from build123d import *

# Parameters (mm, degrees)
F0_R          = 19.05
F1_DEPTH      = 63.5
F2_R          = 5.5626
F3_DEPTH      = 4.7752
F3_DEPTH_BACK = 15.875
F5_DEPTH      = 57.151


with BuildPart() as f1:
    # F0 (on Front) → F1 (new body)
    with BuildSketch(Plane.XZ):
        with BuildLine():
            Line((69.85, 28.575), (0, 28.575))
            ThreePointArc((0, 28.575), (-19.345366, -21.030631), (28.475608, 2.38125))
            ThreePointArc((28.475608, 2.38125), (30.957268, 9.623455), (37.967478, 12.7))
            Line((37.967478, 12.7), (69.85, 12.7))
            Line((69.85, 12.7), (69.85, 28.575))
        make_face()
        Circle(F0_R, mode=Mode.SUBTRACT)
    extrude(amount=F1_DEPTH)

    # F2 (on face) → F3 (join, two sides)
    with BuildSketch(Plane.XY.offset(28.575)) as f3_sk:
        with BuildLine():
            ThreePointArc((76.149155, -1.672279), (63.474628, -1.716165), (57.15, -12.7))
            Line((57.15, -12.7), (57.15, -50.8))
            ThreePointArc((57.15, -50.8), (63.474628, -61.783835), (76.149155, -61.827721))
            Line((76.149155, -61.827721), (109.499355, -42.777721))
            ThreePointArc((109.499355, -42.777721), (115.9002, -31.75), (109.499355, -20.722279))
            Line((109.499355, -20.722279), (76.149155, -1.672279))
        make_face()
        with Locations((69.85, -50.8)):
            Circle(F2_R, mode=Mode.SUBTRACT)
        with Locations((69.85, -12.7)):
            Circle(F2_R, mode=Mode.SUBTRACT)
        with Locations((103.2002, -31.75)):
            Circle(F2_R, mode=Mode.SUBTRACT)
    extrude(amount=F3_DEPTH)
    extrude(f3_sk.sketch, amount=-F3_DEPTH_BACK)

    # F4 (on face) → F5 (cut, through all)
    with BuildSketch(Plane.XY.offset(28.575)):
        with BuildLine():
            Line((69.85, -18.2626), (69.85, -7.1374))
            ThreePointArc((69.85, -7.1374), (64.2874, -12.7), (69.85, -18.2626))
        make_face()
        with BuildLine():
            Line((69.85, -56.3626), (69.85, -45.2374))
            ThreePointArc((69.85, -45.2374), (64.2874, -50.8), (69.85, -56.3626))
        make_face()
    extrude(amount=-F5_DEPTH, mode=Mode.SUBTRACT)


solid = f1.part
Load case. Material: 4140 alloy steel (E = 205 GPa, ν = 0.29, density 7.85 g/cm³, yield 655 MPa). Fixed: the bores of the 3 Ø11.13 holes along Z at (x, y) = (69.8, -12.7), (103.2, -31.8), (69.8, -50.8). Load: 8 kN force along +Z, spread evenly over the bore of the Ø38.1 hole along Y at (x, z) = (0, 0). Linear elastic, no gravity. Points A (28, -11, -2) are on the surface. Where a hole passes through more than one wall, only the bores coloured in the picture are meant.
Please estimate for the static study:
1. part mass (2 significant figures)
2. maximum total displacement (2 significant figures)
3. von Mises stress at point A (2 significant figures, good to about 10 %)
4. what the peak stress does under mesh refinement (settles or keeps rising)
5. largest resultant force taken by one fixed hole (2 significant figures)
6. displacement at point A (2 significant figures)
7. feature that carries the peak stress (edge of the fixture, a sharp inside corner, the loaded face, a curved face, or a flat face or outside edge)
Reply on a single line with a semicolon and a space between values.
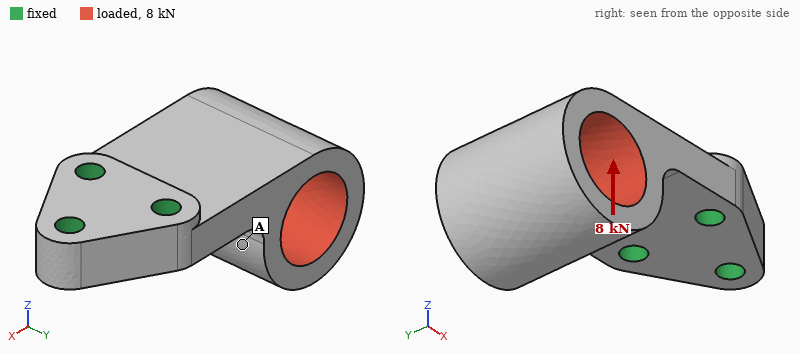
1.4 kg; 0.29 mm; 23 MPa; keeps rising; 5.0 kN; 0.100 mm; edge of the fixture
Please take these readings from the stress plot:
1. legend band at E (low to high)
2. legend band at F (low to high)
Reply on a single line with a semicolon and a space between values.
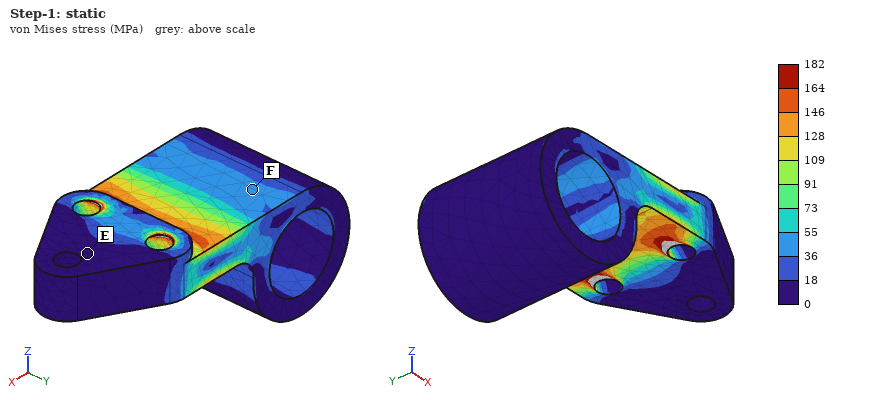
0 to 18 MPa; 36 to 55 MPa
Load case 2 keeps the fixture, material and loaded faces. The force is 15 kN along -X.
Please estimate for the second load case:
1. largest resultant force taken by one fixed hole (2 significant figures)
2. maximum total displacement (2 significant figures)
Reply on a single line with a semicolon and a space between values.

7.1 kN; 0.25 mm
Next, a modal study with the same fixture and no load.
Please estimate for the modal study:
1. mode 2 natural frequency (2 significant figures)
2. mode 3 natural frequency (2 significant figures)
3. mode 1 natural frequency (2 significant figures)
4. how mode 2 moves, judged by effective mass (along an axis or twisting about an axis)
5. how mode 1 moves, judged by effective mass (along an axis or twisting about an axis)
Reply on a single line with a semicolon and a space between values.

2500 Hz; 4400 Hz; 1100 Hz; along Y; along Z
